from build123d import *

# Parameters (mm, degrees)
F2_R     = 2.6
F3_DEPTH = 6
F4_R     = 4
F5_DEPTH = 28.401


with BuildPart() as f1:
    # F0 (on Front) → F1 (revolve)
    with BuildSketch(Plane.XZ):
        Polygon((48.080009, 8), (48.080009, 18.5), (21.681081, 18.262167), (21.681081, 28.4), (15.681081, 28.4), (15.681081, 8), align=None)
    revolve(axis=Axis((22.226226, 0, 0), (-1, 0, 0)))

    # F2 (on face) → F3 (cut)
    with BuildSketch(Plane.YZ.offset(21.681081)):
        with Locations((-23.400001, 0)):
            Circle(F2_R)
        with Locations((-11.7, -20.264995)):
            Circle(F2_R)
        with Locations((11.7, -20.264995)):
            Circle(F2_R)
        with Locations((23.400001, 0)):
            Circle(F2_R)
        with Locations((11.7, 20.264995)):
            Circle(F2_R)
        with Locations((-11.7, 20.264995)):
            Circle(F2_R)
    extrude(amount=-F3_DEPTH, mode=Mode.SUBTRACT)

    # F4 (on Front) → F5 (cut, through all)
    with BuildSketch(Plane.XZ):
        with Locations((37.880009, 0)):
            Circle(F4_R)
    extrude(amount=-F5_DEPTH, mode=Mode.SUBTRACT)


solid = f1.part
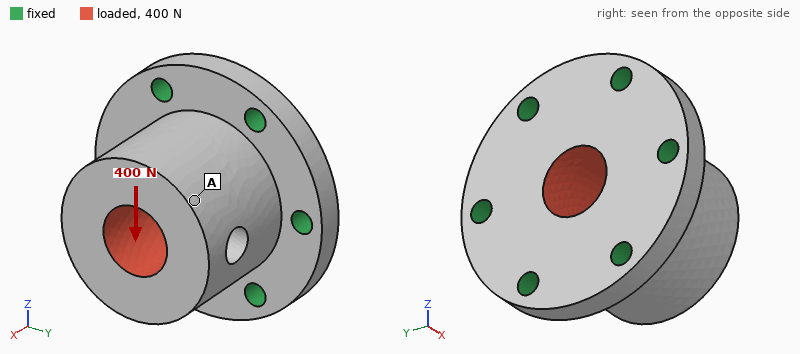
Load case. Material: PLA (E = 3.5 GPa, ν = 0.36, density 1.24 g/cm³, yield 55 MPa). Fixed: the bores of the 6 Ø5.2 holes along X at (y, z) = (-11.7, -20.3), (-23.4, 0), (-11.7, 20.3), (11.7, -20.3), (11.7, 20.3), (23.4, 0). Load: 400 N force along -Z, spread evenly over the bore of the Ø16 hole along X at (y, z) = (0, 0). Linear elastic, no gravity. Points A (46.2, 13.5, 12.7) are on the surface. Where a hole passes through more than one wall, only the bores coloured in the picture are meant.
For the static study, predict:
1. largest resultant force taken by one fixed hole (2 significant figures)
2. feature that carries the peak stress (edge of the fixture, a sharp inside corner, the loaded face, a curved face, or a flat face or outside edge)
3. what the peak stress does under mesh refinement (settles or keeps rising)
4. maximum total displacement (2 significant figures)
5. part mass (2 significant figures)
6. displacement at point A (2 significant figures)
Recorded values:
110 N
edge of the fixture
keeps rising
22 µm
44 g
19 µm
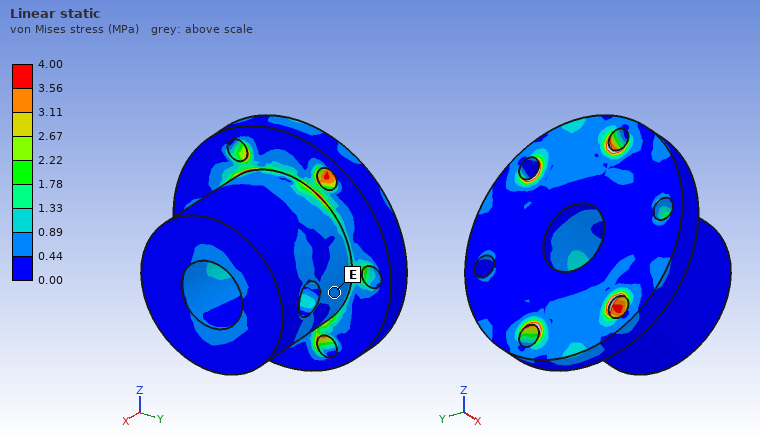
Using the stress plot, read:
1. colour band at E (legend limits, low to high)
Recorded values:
0.44 to 0.89 MPa
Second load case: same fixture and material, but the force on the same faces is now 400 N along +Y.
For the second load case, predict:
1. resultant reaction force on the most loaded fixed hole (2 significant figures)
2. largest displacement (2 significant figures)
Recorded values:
130 N
21 µm
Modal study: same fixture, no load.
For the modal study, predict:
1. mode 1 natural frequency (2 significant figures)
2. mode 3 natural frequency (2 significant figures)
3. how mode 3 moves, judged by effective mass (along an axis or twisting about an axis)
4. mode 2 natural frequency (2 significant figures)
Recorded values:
4300 Hz
6400 Hz
along X
4400 Hz
